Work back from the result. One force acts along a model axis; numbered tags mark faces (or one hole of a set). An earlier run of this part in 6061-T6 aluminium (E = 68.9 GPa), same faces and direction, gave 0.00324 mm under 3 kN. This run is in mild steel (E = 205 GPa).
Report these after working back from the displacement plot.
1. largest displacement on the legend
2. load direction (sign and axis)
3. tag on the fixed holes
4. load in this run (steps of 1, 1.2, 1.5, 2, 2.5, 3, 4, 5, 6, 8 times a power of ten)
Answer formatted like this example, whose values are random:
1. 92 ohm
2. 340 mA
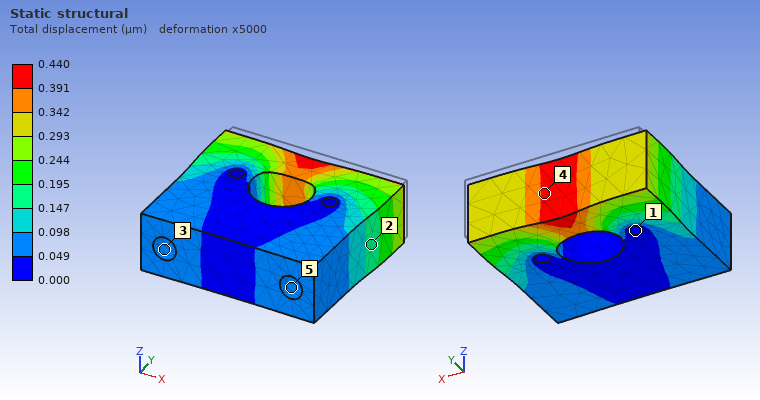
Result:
1. 0.440 µm
2. -Y
3. 1
4. 1.2 kN
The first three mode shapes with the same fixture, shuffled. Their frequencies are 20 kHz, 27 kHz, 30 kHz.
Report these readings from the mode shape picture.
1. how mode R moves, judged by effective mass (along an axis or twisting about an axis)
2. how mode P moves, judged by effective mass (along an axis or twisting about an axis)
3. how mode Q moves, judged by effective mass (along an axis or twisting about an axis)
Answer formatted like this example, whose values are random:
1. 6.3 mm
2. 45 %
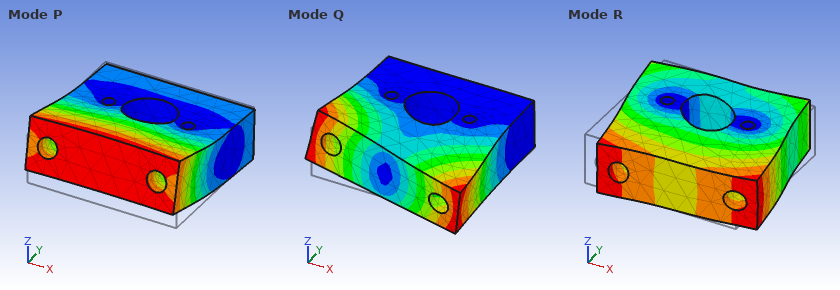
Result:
1. along X
2. along Z
3. twisting about Y
